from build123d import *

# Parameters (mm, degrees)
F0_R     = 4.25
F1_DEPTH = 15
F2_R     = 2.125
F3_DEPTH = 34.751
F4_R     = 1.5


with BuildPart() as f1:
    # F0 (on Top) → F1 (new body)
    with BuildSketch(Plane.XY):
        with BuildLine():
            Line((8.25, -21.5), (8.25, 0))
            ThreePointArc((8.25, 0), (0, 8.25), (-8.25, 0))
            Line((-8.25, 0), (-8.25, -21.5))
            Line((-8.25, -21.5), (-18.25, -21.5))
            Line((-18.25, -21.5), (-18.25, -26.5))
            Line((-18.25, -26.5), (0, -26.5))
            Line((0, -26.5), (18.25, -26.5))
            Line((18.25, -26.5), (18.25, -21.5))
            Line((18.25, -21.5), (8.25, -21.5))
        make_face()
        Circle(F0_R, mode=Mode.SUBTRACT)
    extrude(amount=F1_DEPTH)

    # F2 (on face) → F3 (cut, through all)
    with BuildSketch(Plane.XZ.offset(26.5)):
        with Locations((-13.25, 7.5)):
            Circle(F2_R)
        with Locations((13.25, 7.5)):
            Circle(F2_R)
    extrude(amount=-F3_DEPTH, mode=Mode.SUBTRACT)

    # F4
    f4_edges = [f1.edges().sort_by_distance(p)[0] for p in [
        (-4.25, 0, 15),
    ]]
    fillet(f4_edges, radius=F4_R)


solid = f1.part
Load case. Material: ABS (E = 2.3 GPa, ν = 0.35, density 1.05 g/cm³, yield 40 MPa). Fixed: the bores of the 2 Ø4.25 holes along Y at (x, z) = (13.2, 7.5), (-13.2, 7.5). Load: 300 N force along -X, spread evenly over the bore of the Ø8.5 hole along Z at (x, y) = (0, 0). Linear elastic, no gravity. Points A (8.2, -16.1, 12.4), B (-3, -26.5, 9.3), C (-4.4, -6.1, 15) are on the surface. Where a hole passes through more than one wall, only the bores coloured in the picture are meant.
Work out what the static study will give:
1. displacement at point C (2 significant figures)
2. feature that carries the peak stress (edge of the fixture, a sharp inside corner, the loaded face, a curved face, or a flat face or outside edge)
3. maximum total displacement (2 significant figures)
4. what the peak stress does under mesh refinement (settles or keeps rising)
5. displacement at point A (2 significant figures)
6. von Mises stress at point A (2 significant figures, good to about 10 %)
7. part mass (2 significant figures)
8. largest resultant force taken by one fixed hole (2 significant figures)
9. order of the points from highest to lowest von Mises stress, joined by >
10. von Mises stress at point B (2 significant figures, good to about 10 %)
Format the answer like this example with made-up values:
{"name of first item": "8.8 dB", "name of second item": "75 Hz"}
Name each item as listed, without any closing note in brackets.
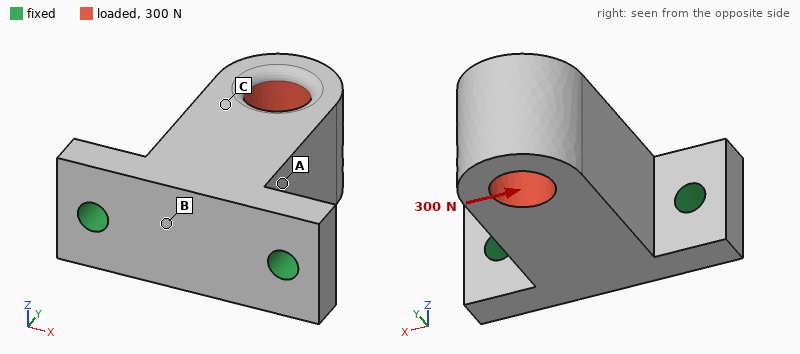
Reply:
{"displacement at point C": "0.18 mm", "feature that carries the peak stress": "edge of the fixture", "maximum total displacement": "0.40 mm", "what the peak stress does under mesh refinement": "keeps rising", "displacement at point A": "0.099 mm", "von Mises stress at point A": "7.1 MPa", "part mass": "9.1 g", "largest resultant force taken by one fixed hole": "370 N", "order of the points from highest to lowest von Mises stress, joined by >": "A > B > C", "von Mises stress at point B": "4.6 MPa"}
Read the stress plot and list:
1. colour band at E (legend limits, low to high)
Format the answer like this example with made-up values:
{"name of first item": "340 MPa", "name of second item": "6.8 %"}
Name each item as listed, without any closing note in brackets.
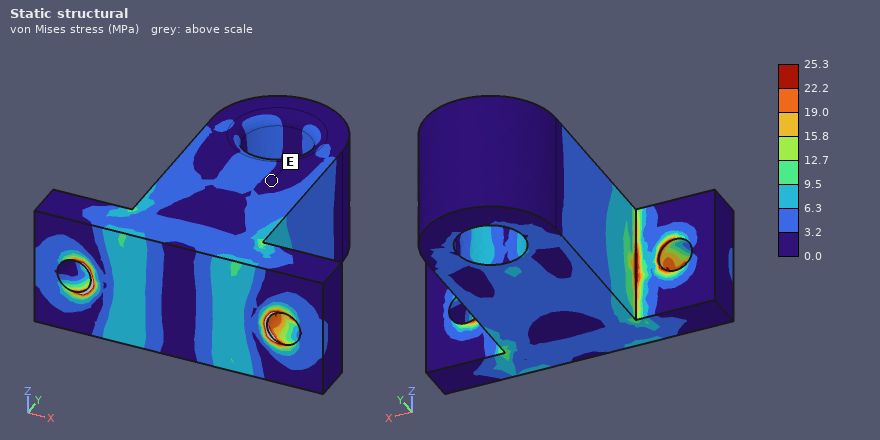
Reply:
{"colour band at E": "0.0 to 3.2 MPa"}
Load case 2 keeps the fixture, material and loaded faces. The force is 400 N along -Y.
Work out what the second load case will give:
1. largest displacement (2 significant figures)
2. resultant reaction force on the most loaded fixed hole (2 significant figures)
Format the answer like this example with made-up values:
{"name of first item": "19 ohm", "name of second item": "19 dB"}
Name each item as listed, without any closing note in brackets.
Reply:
{"largest displacement": "0.11 mm", "resultant reaction force on the most loaded fixed hole": "210 N"}
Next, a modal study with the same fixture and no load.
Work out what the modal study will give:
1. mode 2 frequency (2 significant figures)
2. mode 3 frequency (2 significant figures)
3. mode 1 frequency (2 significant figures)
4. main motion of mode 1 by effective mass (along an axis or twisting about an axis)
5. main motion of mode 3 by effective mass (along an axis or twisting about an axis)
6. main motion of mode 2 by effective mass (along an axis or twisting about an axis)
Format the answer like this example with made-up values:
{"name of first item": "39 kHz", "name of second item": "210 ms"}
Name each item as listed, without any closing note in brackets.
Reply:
{"mode 2 frequency": "2800 Hz", "mode 3 frequency": "5300 Hz", "mode 1 frequency": "1400 Hz", "main motion of mode 1 by effective mass": "along Z", "main motion of mode 3 by effective mass": "along Y", "main motion of mode 2 by effective mass": "along X"}
